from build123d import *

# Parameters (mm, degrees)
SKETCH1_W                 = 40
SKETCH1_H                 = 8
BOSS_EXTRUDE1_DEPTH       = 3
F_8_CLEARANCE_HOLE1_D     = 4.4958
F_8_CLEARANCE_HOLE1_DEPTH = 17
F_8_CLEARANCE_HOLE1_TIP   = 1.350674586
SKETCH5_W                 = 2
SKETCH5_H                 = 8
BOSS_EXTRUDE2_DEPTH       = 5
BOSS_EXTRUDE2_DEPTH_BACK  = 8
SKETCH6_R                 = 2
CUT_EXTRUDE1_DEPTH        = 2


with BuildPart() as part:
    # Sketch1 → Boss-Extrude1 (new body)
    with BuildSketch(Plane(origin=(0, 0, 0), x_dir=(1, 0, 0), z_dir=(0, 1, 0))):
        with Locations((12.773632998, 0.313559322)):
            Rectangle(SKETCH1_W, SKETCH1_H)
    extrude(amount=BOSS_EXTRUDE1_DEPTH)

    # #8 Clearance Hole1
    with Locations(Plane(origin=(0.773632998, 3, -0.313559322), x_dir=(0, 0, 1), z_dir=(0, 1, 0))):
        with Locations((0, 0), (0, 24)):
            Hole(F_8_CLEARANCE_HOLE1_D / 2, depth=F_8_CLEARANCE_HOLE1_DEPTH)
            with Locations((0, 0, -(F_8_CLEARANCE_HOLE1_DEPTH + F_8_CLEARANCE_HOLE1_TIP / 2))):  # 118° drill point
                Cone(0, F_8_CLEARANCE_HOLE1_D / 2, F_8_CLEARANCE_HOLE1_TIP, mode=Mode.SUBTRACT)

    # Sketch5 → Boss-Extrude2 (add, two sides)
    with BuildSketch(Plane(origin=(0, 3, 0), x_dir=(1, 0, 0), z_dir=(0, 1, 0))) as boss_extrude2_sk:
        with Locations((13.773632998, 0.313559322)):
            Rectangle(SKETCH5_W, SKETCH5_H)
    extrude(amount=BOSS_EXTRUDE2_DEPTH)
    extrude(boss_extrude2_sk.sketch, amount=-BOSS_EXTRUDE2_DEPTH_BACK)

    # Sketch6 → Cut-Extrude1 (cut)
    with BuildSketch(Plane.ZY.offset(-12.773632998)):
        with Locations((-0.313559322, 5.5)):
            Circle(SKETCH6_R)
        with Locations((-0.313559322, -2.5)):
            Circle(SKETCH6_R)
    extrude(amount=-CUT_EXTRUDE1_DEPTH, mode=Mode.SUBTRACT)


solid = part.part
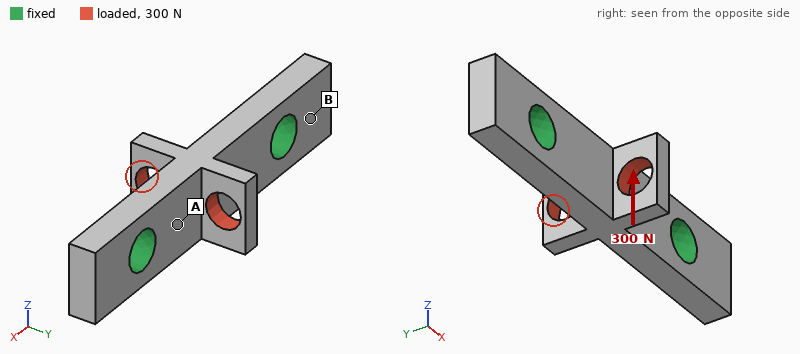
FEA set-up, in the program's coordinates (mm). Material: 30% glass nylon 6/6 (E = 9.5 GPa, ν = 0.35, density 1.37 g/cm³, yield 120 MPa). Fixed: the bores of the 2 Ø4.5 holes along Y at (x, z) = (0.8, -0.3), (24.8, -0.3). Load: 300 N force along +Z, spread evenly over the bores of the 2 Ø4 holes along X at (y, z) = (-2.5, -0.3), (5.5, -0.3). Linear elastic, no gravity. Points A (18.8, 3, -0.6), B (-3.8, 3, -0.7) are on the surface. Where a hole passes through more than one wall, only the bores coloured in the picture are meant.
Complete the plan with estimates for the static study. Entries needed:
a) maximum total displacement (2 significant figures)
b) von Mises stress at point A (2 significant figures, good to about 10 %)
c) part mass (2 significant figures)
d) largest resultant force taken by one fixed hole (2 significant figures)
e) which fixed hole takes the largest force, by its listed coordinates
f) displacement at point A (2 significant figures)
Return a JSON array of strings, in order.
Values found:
["95 µm", "19 MPa", "1.3 g", "170 N", "(24.8, -0.3)", "18 µm"]
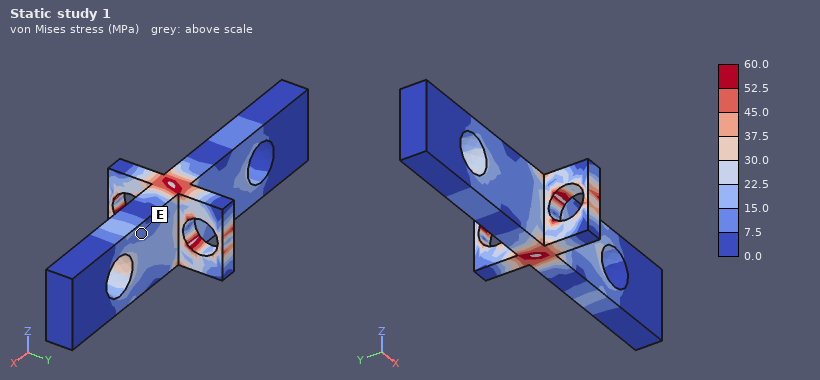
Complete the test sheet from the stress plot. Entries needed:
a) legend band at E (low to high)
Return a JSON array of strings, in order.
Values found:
["7.5 to 15.0 MPa"]
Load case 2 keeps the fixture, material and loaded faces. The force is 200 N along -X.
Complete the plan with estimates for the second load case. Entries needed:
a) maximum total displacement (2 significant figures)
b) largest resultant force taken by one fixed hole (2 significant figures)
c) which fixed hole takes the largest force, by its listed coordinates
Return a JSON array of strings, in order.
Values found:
["98 µm", "110 N", "(24.8, -0.3)"]
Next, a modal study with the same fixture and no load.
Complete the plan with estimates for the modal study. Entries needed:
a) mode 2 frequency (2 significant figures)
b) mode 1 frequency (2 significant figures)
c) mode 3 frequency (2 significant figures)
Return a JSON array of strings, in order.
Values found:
["14 kHz", "14 kHz", "20 kHz"]
